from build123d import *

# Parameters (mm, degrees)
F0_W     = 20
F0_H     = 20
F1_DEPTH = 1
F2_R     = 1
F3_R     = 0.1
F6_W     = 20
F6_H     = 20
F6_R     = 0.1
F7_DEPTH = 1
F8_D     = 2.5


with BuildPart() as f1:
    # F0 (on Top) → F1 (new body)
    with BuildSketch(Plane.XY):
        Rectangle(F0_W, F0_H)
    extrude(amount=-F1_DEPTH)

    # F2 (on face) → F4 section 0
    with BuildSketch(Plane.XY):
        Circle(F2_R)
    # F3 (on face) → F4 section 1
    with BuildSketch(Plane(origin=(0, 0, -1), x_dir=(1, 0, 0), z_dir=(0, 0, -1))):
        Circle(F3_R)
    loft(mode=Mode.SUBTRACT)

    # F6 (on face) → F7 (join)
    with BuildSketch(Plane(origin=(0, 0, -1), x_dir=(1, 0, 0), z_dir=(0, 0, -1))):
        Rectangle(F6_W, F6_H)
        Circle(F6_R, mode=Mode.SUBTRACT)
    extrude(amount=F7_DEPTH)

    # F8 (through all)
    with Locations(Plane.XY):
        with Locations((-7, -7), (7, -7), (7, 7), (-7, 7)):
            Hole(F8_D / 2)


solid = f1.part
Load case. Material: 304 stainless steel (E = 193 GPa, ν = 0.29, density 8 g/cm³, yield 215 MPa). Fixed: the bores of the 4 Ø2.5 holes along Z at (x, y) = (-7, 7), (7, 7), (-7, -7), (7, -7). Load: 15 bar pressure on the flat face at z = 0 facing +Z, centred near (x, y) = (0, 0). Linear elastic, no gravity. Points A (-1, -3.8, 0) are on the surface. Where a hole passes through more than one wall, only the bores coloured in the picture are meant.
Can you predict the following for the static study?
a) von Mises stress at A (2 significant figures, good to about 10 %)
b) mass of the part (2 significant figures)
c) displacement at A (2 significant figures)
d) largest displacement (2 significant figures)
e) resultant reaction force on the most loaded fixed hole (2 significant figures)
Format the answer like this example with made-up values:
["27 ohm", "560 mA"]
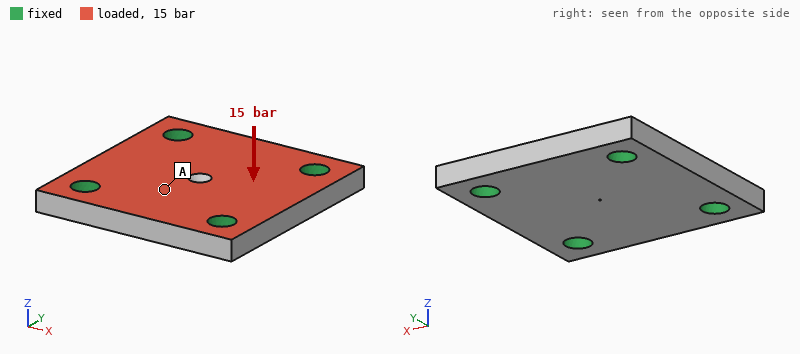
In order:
["14 MPa", "6.1 g", "1.8 µm", "2.3 µm", "140 N"]
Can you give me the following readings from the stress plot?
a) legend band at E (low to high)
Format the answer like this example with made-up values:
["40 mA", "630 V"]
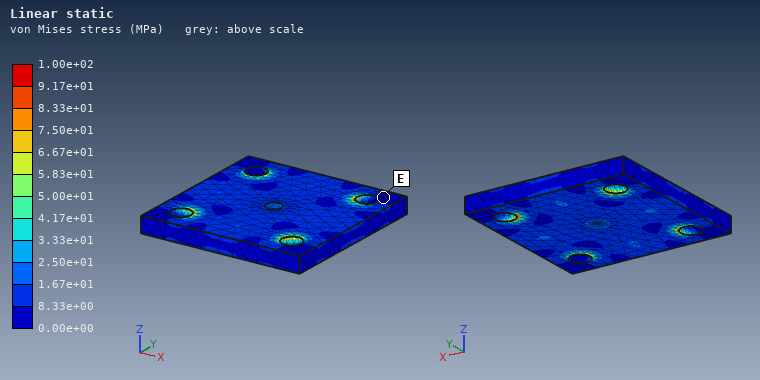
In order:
["0.00e+00 to 8.33e+00 MPa"]
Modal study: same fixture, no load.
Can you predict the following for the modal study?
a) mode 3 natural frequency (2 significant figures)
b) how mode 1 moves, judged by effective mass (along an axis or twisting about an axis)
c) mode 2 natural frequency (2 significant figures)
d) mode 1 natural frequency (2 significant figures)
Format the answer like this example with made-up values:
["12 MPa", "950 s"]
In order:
["58 kHz", "along Z", "58 kHz", "39 kHz"]
